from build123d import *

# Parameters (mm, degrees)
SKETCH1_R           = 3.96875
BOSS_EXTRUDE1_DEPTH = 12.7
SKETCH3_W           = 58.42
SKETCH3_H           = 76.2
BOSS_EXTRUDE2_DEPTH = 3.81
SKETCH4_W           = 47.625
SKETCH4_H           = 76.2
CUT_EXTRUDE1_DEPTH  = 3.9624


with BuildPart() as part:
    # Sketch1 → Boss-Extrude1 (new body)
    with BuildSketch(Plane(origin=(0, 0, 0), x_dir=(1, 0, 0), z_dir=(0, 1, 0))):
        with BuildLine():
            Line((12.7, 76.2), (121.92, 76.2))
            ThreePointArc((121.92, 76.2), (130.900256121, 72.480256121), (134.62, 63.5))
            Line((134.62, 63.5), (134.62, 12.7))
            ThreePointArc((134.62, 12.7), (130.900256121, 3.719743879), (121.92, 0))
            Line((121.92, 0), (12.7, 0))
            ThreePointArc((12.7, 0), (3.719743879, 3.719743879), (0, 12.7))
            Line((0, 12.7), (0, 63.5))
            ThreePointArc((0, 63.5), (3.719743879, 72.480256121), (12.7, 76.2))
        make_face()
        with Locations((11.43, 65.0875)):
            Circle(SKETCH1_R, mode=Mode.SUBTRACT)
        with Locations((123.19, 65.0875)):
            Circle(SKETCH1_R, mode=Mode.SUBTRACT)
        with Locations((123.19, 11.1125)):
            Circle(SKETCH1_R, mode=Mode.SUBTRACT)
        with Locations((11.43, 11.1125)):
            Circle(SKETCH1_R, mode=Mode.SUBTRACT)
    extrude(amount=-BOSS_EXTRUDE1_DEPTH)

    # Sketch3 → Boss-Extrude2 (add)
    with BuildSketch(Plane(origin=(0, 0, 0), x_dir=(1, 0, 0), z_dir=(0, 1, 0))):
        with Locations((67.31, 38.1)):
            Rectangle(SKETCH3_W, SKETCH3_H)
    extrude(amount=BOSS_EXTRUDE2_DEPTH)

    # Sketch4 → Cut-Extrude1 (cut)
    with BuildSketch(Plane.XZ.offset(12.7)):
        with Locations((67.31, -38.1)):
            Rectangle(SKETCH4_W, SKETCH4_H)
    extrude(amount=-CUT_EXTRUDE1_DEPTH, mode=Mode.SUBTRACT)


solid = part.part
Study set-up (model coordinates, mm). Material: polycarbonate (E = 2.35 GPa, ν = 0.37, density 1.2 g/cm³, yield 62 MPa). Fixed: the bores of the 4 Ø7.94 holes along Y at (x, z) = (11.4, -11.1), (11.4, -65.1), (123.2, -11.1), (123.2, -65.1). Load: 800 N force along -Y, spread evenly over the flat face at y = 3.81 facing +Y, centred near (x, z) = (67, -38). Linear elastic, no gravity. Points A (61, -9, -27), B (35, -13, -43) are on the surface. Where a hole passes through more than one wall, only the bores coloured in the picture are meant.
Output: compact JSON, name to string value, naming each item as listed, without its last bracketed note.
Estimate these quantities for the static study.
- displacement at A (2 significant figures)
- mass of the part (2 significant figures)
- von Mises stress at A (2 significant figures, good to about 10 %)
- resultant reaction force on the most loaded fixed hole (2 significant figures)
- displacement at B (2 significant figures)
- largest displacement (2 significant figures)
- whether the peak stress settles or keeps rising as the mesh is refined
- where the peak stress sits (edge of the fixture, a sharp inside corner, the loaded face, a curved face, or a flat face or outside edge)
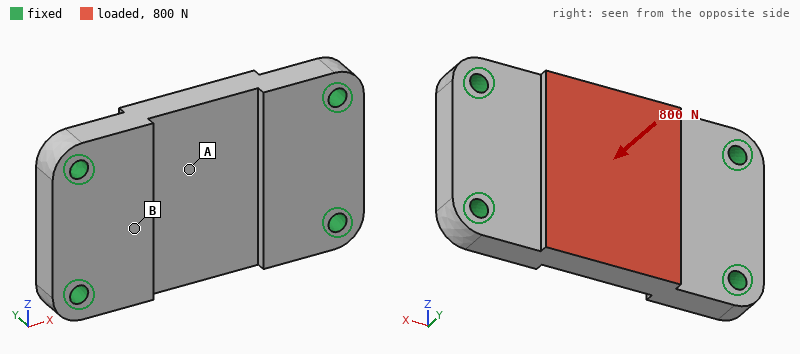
{"displacement at A": "0.16 mm", "mass of the part": "150 g", "von Mises stress at A": "1.9 MPa", "resultant reaction force on the most loaded fixed hole": "320 N", "displacement at B": "0.092 mm", "largest displacement": "0.18 mm", "whether the peak stress settles or keeps rising as the mesh is refined": "keeps rising", "where the peak stress sits": "edge of the fixture"}
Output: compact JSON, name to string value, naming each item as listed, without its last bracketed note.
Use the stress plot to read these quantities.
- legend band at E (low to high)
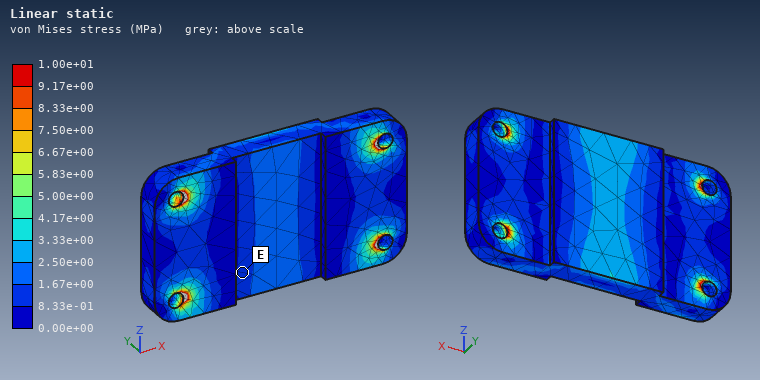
{"legend band at E": "8.33e-01 to 1.67e+00 MPa"}
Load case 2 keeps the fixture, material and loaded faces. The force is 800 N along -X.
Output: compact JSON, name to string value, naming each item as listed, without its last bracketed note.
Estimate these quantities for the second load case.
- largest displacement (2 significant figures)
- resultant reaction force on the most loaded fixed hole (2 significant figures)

{"largest displacement": "14 µm", "resultant reaction force on the most loaded fixed hole": "210 N"}
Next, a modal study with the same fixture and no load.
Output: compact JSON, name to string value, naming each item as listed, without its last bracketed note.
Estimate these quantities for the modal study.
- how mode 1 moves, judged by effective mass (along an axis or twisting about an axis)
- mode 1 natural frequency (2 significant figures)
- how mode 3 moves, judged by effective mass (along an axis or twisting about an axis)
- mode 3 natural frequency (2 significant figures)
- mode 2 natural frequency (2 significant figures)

{"how mode 1 moves, judged by effective mass": "along Y", "mode 1 natural frequency": "1300 Hz", "how mode 3 moves, judged by effective mass": "twisting about Z", "mode 3 natural frequency": "3100 Hz", "mode 2 natural frequency": "1900 Hz"}
